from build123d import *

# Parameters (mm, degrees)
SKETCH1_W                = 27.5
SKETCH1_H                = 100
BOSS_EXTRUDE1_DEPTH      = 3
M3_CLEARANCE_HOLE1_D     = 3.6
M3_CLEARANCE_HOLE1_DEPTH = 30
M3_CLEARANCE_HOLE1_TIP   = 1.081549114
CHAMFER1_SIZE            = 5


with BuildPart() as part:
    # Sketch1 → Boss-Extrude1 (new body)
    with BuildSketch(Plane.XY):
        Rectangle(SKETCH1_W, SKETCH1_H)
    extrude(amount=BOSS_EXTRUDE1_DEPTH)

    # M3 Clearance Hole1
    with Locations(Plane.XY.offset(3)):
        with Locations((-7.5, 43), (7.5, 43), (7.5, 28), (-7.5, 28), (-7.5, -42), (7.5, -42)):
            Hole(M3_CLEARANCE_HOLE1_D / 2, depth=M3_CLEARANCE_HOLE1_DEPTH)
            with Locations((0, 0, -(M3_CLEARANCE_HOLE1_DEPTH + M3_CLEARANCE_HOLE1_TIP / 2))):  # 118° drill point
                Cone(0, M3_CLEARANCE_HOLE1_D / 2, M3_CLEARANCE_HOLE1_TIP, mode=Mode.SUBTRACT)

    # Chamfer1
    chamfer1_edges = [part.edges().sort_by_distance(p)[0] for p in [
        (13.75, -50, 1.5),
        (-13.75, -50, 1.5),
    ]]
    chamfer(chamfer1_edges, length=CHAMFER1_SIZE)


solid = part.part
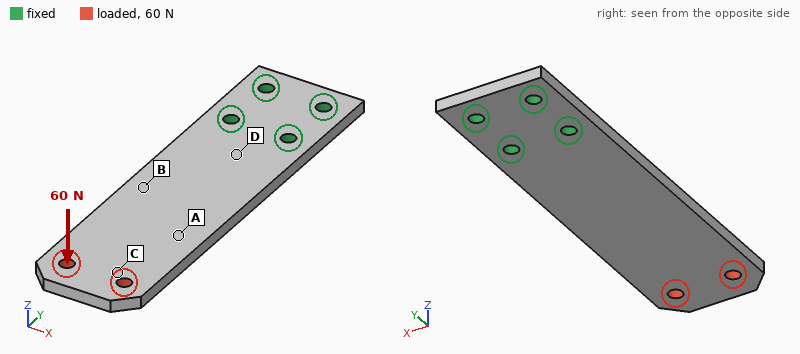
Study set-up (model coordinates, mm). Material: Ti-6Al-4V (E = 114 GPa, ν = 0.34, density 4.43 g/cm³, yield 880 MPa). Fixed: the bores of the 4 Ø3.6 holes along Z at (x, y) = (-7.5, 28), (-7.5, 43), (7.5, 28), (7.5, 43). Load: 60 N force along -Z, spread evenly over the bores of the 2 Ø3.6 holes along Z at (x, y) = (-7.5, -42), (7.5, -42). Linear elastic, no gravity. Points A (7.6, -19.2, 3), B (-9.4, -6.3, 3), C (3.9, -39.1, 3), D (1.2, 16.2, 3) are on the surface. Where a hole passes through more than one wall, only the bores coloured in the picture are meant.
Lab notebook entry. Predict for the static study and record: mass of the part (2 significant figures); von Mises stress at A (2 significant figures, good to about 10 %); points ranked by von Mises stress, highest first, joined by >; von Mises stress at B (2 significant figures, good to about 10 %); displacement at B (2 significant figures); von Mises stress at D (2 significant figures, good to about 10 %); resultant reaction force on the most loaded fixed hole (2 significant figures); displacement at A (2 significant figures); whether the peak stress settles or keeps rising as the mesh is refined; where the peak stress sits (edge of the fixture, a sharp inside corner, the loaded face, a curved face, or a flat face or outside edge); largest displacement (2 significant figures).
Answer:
35 g
33 MPa
D > B > A > C
52 MPa
0.27 mm
78 MPa
51 N
0.49 mm
keeps rising
edge of the fixture
1.1 mm
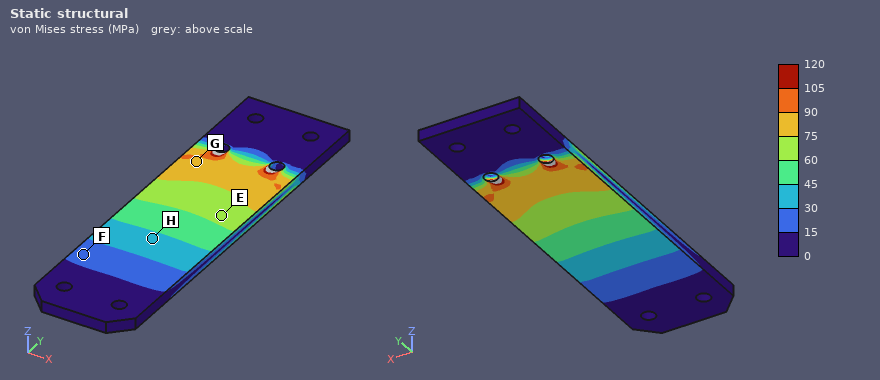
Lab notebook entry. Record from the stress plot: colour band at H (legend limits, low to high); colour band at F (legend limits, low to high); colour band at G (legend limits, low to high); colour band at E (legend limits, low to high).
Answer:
30 to 45 MPa
15 to 30 MPa
75 to 90 MPa
60 to 75 MPa
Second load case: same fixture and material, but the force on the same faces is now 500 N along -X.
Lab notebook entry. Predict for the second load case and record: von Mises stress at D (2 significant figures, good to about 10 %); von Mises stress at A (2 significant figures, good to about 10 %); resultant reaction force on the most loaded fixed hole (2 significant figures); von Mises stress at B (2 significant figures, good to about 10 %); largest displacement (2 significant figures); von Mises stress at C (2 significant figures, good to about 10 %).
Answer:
21 MPa
20 MPa
1.7 kN
33 MPa
0.13 mm
12 MPa
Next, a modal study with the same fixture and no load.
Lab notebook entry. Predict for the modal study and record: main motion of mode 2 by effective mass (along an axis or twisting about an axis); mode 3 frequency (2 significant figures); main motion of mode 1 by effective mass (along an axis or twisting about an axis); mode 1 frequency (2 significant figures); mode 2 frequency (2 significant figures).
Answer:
twisting about Y
2600 Hz
along Z
430 Hz
2400 Hz
